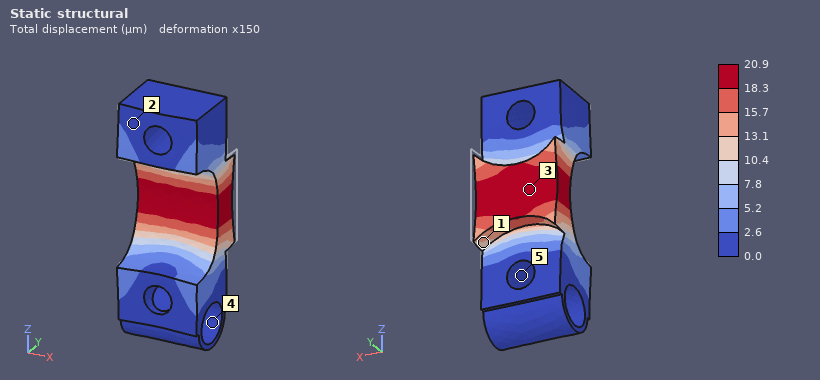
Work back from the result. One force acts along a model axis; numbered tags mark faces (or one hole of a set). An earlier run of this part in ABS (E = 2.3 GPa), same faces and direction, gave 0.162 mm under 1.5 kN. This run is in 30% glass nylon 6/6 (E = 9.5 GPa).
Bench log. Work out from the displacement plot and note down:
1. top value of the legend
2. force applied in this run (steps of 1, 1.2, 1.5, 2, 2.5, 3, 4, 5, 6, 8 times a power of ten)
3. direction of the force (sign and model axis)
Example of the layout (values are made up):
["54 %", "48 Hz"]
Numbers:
["20.9 µm", "800 N", "-Y"]
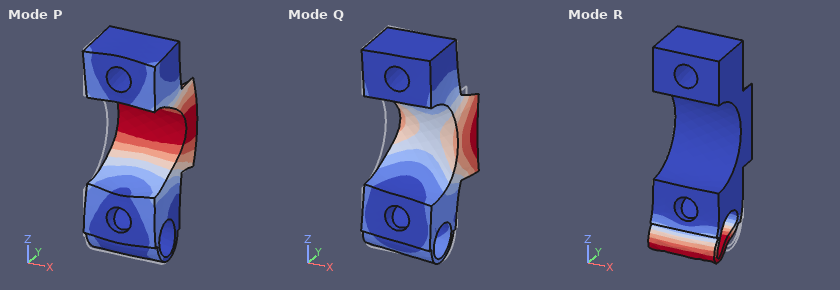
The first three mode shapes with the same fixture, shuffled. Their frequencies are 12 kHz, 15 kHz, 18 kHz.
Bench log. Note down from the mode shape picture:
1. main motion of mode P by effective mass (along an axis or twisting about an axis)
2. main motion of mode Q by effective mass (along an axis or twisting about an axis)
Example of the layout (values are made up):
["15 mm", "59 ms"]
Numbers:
["along Y", "along X"]
